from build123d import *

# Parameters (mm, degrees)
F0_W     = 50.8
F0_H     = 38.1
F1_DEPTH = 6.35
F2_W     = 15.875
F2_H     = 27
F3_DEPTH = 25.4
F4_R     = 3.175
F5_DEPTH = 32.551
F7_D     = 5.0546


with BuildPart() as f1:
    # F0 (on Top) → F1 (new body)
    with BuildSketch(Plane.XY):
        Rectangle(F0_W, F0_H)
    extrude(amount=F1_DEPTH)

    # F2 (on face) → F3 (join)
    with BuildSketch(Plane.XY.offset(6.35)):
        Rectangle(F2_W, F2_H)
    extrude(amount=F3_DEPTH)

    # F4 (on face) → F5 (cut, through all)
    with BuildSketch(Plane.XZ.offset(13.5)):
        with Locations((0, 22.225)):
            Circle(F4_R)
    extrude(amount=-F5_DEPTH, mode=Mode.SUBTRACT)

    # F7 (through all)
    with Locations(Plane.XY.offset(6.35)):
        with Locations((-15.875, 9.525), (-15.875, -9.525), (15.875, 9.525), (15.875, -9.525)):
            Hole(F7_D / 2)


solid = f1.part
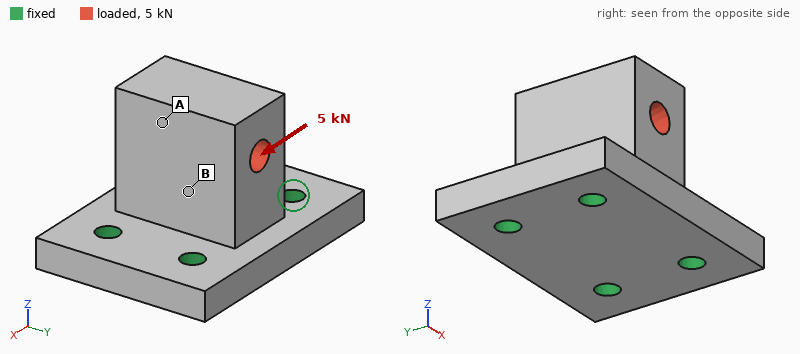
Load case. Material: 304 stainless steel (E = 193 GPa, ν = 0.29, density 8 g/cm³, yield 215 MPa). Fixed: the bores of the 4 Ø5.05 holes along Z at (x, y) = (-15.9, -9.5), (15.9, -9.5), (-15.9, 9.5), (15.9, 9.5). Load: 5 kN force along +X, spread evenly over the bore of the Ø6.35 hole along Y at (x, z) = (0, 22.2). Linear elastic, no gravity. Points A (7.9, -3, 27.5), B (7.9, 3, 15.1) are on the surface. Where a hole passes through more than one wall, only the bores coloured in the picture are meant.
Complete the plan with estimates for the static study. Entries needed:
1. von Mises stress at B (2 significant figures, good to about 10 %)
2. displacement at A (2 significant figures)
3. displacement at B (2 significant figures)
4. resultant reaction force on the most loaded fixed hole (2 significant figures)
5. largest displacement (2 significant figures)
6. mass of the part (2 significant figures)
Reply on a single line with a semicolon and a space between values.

34 MPa; 22 µm; 11 µm; 2.4 kN; 26 µm; 170 g
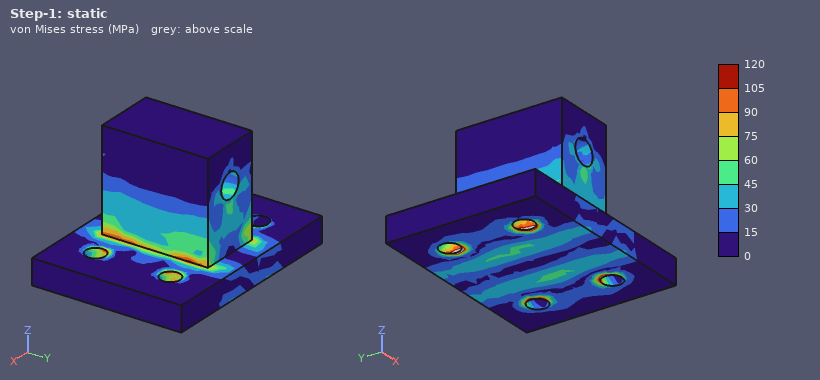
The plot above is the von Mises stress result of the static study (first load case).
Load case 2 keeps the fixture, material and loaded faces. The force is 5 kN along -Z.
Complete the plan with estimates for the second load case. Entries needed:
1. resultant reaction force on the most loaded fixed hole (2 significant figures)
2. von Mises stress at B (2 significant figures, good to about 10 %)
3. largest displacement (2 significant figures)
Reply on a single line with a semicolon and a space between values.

1.3 kN; 11 MPa; 4.9 µm
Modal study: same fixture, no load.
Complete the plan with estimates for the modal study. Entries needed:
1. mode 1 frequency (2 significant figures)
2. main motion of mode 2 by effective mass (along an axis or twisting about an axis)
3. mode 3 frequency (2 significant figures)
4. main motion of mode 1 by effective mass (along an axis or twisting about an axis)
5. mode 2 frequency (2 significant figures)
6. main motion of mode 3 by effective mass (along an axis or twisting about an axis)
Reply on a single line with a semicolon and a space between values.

9900 Hz; along X; 17 kHz; along Y; 10 kHz; along Z
